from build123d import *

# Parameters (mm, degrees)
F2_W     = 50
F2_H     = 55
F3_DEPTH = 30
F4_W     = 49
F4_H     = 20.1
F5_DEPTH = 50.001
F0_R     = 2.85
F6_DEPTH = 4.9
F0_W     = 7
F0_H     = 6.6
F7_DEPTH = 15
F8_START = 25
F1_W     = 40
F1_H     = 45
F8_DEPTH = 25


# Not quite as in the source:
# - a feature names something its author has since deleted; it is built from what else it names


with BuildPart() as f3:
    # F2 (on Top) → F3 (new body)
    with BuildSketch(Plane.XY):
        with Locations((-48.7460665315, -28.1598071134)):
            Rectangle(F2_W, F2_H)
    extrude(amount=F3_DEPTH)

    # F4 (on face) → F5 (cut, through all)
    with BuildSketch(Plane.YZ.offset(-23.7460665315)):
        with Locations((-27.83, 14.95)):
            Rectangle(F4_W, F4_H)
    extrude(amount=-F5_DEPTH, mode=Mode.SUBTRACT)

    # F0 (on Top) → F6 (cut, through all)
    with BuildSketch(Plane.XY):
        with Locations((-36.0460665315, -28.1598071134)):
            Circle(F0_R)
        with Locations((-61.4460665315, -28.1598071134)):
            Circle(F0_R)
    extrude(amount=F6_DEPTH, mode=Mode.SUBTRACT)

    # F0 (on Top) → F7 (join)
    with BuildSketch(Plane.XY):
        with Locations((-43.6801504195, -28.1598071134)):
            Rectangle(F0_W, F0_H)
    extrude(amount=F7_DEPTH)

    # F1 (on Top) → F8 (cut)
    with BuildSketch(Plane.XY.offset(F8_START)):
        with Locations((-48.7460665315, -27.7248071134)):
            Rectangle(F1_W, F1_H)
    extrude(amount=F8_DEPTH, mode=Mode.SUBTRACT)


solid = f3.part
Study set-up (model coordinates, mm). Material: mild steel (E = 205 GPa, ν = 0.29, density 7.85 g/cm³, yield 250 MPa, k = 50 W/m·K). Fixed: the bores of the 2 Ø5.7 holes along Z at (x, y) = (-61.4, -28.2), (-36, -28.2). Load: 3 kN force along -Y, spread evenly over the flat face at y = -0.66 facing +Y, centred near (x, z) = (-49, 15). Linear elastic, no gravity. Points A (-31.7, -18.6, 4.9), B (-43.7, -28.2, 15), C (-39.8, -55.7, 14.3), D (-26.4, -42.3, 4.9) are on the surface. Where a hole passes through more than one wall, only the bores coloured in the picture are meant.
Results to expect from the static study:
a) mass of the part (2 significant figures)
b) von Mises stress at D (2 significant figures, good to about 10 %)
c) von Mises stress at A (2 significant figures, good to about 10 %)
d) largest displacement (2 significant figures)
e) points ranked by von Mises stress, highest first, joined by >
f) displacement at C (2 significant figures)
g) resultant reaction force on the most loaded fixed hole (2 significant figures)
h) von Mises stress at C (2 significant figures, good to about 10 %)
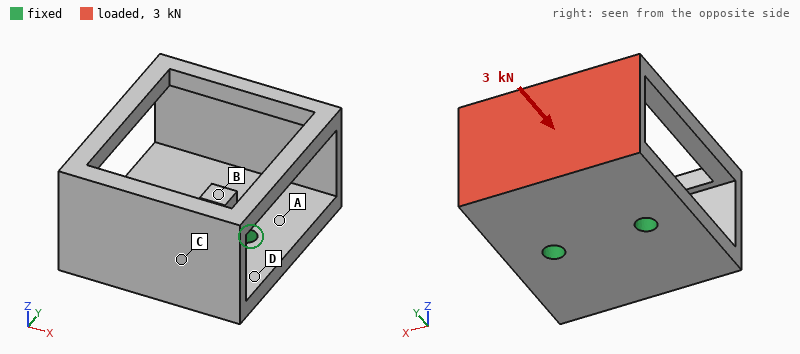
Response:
190 g
73 MPa
98 MPa
0.20 mm
A > D > C > B
0.081 mm
1.5 kN
39 MPa
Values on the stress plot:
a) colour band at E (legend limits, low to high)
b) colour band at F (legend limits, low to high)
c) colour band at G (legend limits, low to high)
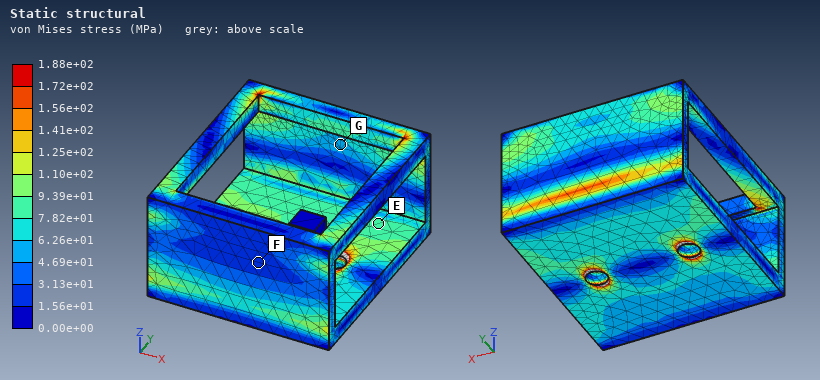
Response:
7.82e+01 to 9.39e+01 MPa
1.56e+01 to 3.13e+01 MPa
4.69e+01 to 6.26e+01 MPa
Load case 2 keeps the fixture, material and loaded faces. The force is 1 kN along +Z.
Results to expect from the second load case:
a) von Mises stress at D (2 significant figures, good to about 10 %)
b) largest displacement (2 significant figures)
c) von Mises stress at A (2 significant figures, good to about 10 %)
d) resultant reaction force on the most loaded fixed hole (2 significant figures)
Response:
17 MPa
71 µm
66 MPa
510 N
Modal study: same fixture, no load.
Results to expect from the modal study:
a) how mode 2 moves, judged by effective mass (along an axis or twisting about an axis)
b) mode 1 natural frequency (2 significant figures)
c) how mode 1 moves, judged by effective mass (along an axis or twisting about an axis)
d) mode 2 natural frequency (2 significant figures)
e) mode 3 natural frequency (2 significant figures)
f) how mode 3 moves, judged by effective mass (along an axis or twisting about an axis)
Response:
along X
1900 Hz
along Y
3000 Hz
3400 Hz
along Z
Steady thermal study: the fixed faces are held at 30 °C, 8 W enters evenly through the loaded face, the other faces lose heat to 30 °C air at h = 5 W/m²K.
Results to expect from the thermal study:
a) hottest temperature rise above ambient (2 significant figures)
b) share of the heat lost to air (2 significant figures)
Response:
26 K
6.5 %
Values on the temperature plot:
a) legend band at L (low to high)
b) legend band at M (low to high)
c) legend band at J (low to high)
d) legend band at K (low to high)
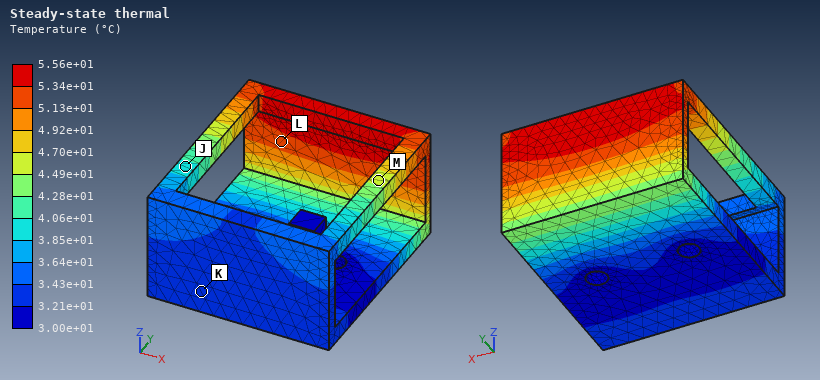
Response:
5.13e+01 to 5.34e+01 °C
4.49e+01 to 4.70e+01 °C
3.85e+01 to 4.06e+01 °C
3.21e+01 to 3.43e+01 °C
